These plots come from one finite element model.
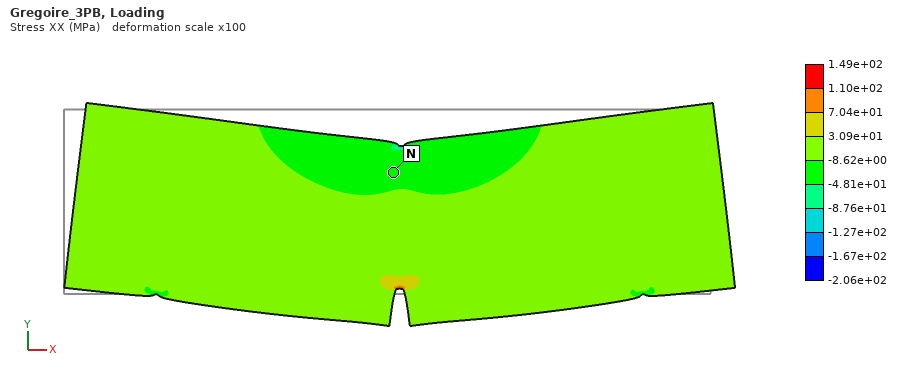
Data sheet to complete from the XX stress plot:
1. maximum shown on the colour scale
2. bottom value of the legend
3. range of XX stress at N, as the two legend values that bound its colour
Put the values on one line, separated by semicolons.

1.49e+02 MPa; -2.06e+02 MPa; -4.81e+01 to -8.62e+00 MPa
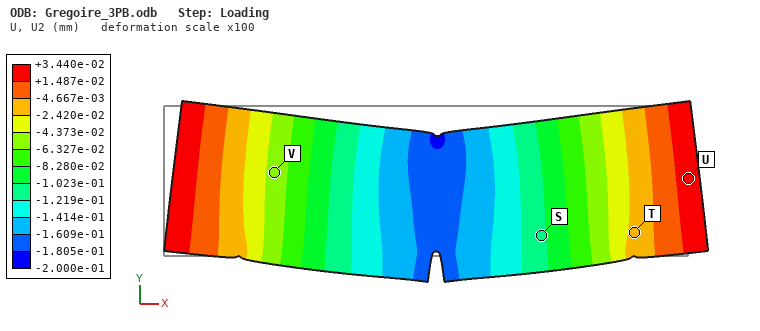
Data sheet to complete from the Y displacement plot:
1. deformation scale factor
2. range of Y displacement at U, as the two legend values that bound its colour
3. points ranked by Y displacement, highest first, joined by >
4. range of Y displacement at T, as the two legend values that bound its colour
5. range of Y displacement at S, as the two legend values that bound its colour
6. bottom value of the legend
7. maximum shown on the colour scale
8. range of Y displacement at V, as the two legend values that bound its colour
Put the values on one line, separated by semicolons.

100; +1.487e-02 to +3.440e-02 mm; U > T > V > S; -2.420e-02 to -4.667e-03 mm; -1.219e-01 to -1.023e-01 mm; -2.000e-01 mm; +3.440e-02 mm; -6.327e-02 to -4.373e-02 mm
